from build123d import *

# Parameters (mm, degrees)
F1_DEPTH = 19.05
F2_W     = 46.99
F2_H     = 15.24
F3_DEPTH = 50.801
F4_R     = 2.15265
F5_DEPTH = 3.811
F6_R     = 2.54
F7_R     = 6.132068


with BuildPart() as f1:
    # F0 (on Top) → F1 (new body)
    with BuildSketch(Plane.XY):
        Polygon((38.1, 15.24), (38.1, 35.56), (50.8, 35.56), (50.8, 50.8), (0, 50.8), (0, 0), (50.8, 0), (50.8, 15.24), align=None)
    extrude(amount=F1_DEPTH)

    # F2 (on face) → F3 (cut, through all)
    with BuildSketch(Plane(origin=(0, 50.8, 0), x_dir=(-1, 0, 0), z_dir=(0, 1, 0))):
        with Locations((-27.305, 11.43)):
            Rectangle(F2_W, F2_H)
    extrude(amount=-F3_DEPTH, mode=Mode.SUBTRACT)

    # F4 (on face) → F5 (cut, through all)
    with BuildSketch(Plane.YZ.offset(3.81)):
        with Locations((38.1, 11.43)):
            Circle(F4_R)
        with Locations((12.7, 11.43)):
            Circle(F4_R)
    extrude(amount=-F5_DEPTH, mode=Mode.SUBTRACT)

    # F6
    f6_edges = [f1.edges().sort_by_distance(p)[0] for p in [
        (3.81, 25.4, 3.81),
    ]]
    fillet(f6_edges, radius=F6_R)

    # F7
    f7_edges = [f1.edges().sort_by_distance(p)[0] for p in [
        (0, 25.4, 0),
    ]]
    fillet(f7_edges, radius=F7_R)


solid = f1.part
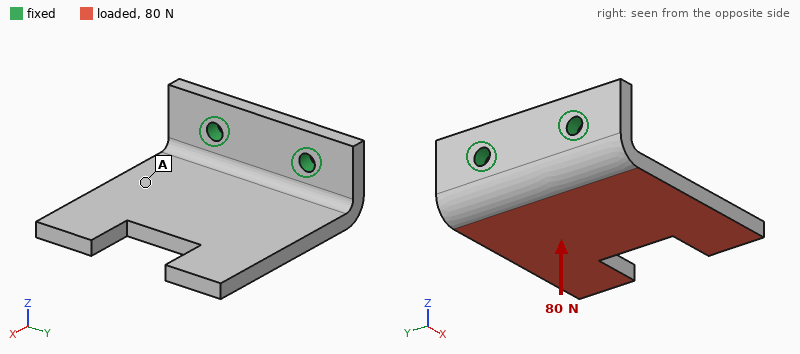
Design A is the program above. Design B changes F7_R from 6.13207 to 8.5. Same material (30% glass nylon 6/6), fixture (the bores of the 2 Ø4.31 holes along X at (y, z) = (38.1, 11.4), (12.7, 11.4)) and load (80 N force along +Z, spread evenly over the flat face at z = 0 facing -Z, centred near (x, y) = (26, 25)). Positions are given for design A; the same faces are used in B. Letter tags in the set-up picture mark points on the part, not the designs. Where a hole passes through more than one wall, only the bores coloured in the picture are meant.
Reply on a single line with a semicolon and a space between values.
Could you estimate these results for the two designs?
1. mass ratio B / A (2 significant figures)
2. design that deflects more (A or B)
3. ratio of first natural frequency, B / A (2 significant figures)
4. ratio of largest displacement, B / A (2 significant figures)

0.97; B; 0.89; 1.3
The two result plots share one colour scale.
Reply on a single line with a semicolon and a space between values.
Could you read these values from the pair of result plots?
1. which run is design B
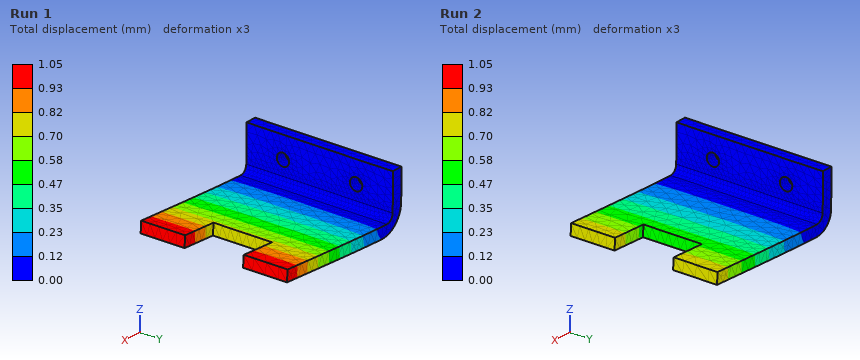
Run 1
